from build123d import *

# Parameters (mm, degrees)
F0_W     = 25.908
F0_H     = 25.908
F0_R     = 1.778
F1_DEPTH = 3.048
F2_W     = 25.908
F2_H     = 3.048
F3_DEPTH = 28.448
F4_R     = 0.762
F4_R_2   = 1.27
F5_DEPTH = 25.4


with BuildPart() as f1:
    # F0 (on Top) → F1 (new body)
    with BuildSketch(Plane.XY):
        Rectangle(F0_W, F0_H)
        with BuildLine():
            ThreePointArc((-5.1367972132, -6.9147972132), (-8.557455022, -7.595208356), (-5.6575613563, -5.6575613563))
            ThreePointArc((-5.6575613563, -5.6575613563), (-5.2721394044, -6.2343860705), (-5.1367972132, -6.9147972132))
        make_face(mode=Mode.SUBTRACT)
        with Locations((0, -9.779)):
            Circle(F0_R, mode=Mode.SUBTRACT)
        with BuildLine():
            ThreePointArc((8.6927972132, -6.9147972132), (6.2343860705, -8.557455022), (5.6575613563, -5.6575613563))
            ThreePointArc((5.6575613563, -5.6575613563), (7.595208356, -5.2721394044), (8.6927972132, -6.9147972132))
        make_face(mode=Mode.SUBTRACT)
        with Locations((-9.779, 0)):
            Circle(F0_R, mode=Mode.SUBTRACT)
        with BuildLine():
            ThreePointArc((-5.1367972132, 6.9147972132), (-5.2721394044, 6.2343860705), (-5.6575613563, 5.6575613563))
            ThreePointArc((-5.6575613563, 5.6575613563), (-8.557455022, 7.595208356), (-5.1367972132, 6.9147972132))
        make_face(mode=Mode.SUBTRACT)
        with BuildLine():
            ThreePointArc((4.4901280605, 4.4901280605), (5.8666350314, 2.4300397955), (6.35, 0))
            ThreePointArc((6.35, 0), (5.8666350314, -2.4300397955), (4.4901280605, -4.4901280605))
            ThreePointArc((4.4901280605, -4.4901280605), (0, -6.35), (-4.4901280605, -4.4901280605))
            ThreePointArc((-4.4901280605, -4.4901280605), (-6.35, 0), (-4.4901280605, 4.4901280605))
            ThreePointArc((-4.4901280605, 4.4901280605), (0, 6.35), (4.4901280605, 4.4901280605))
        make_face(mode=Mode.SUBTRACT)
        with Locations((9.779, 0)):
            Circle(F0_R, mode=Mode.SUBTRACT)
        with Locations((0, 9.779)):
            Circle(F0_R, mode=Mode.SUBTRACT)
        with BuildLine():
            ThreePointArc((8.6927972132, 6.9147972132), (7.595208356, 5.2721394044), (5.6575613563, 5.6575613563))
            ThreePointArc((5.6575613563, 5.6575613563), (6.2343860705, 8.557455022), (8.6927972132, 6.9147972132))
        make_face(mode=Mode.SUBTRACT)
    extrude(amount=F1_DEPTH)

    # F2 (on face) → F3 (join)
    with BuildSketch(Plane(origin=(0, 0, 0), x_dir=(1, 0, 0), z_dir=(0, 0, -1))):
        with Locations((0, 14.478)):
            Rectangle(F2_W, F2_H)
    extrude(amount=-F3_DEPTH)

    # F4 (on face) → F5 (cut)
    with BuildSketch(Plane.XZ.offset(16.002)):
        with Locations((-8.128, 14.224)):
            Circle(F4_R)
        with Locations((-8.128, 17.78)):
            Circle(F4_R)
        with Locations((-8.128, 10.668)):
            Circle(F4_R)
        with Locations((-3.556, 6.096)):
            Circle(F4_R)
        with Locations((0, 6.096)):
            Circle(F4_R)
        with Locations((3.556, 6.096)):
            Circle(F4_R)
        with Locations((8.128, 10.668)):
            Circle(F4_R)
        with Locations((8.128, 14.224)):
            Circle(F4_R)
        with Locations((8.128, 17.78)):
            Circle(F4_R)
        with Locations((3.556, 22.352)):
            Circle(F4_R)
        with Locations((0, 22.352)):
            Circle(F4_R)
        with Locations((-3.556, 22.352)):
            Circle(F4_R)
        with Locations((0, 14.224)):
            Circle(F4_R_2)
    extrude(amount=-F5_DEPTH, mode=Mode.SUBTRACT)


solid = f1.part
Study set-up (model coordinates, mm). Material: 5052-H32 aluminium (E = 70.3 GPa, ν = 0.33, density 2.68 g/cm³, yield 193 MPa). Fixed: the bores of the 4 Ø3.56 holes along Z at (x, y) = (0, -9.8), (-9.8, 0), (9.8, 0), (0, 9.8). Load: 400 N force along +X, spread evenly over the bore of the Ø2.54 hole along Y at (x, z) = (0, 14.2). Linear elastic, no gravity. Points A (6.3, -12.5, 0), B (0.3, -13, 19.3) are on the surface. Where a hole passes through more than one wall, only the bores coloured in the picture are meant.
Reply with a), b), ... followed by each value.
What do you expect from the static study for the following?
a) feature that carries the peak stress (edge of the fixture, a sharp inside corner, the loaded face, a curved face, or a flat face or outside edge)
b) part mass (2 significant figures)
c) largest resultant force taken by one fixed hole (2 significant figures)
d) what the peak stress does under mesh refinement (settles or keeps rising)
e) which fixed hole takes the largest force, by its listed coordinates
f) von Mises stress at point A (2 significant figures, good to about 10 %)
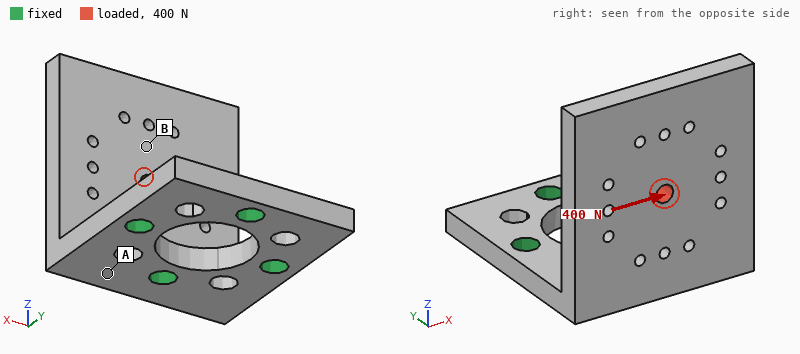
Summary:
a) edge of the fixture
b) 9.6 g
c) 380 N
d) keeps rising
e) (0, -9.8)
f) 27 MPa
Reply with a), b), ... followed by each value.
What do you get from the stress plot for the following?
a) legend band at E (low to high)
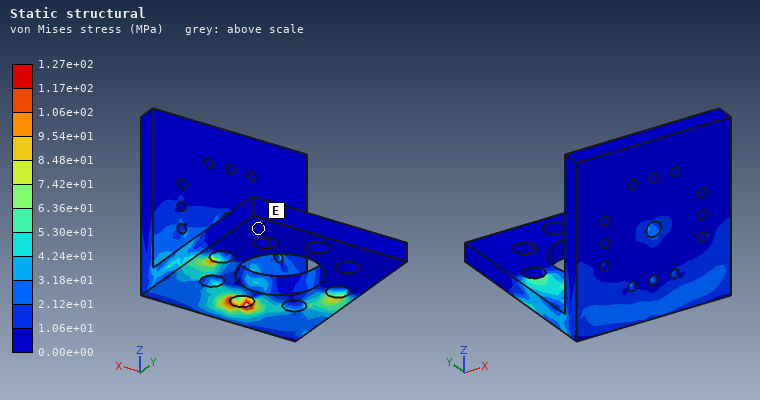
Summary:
a) 0.00e+00 to 1.06e+01 MPa
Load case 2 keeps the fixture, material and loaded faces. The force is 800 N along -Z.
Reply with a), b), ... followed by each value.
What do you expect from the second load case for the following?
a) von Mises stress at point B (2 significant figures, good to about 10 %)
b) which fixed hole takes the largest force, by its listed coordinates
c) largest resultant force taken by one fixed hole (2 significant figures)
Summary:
a) 10 MPa
b) (0, -9.8)
c) 850 N
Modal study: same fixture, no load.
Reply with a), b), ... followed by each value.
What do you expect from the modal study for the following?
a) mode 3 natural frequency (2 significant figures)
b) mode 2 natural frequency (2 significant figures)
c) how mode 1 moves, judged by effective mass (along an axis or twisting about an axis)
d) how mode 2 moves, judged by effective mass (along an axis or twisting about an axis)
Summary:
a) 7800 Hz
b) 4700 Hz
c) along Y
d) along X
